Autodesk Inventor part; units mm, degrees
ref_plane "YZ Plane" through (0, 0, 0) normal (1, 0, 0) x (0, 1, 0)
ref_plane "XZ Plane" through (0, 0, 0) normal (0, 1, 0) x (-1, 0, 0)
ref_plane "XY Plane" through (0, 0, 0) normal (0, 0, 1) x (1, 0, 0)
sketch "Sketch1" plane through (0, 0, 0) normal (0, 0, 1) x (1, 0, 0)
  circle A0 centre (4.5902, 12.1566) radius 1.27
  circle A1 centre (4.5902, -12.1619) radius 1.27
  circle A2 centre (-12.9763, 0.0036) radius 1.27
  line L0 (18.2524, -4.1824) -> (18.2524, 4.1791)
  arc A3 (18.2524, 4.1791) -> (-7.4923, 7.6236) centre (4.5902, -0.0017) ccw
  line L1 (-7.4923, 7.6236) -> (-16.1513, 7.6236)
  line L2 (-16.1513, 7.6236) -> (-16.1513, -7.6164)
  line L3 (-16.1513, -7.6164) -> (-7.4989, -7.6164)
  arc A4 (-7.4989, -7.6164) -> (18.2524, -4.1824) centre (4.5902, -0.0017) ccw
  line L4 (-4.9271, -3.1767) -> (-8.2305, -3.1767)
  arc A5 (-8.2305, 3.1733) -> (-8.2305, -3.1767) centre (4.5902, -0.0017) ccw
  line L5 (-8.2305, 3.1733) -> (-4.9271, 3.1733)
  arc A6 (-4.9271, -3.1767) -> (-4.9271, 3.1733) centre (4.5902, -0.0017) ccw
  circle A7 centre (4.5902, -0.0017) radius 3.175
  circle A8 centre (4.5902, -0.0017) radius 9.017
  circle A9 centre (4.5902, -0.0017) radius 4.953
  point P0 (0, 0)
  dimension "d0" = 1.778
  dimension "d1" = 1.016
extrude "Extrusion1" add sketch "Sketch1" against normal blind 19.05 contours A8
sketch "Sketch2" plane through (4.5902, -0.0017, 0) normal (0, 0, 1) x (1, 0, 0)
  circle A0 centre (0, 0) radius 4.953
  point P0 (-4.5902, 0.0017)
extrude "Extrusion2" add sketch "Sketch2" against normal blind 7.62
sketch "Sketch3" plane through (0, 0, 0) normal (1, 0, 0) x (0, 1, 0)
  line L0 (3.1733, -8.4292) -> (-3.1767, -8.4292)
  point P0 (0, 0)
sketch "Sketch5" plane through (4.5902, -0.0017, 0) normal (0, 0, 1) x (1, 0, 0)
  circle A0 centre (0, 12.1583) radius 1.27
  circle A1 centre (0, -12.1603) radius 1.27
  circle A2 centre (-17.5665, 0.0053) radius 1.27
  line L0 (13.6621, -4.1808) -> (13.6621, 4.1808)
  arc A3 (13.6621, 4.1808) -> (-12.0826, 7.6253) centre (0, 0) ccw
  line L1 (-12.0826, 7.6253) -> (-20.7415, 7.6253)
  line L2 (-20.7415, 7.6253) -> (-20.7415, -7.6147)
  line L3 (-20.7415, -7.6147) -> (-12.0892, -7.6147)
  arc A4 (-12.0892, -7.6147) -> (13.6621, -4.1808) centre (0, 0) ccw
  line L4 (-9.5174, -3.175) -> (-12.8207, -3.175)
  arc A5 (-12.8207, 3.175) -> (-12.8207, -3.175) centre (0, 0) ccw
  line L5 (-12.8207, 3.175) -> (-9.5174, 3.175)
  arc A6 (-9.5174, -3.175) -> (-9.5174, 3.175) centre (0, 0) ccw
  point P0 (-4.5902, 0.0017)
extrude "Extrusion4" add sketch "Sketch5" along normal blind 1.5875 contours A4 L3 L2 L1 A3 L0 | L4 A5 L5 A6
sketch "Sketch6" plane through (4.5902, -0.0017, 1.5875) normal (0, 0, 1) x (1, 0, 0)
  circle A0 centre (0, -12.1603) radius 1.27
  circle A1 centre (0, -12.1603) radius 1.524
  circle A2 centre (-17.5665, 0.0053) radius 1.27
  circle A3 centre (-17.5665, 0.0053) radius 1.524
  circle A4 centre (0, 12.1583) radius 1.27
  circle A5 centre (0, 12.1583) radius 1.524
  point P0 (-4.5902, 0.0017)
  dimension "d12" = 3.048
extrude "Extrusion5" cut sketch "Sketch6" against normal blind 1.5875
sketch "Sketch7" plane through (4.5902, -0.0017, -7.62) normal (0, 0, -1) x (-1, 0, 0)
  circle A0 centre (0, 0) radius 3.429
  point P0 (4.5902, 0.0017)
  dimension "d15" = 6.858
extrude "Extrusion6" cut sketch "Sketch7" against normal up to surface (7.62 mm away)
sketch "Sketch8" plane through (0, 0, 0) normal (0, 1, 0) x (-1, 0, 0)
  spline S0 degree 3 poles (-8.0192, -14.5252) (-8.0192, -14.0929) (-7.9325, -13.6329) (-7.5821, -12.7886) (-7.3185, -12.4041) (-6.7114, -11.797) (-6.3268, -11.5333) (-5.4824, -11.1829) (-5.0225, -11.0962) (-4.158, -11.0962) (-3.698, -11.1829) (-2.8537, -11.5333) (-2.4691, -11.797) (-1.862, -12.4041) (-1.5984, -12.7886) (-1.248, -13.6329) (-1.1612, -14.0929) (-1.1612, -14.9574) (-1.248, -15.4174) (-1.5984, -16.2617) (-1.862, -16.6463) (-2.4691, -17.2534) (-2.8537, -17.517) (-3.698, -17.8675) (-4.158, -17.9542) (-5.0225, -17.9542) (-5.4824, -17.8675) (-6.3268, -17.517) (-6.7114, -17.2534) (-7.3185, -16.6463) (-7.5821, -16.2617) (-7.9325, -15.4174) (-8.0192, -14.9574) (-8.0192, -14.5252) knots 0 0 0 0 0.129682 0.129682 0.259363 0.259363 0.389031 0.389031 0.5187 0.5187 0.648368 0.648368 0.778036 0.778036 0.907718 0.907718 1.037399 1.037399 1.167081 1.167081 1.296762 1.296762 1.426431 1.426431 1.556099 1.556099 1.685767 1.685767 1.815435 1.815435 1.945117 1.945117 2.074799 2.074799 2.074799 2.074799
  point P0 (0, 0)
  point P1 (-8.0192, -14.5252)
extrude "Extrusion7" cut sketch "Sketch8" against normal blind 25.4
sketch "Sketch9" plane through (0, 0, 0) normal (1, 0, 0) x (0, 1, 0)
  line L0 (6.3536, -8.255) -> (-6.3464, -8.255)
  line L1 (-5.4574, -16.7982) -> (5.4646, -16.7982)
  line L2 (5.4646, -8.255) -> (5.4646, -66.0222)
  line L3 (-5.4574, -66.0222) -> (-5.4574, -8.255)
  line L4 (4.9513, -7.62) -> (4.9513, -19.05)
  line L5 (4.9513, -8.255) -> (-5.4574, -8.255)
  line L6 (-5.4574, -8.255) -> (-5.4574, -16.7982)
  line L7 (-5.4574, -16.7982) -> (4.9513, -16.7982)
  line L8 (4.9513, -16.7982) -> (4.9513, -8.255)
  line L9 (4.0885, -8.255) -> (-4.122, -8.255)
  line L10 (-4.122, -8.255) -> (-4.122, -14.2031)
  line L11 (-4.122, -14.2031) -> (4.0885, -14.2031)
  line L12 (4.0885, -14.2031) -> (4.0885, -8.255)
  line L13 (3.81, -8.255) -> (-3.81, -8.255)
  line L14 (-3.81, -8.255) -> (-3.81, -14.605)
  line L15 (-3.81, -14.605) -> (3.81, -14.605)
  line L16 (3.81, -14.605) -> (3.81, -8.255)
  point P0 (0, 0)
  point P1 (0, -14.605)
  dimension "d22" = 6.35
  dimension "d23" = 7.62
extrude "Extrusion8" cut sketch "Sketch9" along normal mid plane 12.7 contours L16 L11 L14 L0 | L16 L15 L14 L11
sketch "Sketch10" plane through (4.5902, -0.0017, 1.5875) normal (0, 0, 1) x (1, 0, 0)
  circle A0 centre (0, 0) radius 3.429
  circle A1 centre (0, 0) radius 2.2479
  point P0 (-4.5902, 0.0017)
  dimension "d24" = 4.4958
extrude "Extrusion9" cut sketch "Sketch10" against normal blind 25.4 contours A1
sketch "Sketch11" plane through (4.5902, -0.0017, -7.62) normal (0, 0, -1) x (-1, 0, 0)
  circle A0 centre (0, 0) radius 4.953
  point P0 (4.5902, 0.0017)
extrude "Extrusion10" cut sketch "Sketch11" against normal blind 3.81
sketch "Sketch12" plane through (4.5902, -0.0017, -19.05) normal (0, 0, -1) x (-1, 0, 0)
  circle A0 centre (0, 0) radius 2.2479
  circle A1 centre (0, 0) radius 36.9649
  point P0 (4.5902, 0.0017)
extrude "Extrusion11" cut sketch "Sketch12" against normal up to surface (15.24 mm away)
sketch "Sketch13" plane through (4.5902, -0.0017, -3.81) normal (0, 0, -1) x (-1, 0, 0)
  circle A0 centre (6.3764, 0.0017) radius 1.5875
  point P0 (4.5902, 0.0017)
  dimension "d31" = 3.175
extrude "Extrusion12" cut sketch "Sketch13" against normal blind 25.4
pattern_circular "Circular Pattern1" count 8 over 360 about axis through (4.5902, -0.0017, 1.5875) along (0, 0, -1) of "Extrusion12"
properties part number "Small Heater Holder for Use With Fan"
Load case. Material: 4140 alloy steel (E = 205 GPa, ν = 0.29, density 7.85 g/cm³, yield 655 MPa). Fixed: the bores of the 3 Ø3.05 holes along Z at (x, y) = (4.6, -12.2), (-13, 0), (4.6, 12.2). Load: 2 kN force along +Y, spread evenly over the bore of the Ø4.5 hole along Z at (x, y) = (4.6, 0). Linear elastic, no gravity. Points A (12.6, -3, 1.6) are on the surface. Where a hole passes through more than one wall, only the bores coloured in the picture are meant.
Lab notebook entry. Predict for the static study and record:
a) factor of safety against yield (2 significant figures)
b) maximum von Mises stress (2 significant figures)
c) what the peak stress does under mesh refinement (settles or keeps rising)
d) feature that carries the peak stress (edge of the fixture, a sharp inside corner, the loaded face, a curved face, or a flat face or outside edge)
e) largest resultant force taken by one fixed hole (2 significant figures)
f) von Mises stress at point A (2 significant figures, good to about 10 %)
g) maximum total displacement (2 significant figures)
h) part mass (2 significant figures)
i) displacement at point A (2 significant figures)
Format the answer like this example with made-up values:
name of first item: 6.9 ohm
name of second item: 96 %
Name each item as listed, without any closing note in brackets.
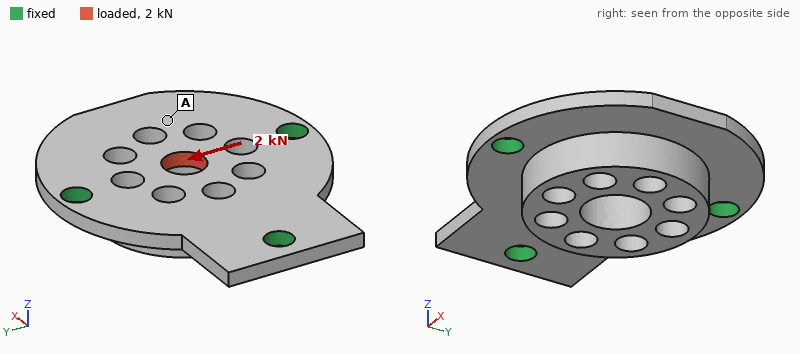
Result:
factor of safety against yield: 2.8
maximum von Mises stress: 230 MPa
what the peak stress does under mesh refinement: settles
feature that carries the peak stress: a curved face
largest resultant force taken by one fixed hole: 910 N
von Mises stress at point A: 18 MPa
maximum total displacement: 5.2 µm
part mass: 13 g
displacement at point A: 3.3 µm
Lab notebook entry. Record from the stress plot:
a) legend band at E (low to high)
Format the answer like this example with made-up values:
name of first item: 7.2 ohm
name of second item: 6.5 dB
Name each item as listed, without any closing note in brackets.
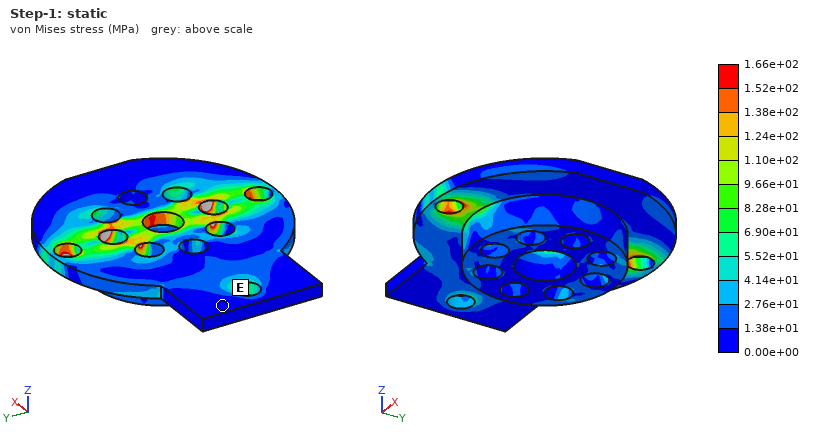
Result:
legend band at E: 0.00e+00 to 1.38e+01 MPa
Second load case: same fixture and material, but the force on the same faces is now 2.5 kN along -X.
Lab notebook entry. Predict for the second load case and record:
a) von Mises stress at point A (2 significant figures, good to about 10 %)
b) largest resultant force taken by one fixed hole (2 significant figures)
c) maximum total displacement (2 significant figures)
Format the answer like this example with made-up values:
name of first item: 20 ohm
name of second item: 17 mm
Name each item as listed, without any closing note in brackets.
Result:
von Mises stress at point A: 57 MPa
largest resultant force taken by one fixed hole: 880 N
maximum total displacement: 7.7 µm
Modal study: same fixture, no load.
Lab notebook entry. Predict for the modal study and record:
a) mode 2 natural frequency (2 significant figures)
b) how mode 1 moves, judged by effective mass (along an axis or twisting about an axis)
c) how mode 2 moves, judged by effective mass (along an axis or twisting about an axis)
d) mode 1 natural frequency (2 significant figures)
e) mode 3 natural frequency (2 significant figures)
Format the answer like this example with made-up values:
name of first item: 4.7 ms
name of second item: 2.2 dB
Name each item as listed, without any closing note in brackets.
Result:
mode 2 natural frequency: 19 kHz
how mode 1 moves, judged by effective mass: along Z
how mode 2 moves, judged by effective mass: along Z
mode 1 natural frequency: 10 kHz
mode 3 natural frequency: 26 kHz
